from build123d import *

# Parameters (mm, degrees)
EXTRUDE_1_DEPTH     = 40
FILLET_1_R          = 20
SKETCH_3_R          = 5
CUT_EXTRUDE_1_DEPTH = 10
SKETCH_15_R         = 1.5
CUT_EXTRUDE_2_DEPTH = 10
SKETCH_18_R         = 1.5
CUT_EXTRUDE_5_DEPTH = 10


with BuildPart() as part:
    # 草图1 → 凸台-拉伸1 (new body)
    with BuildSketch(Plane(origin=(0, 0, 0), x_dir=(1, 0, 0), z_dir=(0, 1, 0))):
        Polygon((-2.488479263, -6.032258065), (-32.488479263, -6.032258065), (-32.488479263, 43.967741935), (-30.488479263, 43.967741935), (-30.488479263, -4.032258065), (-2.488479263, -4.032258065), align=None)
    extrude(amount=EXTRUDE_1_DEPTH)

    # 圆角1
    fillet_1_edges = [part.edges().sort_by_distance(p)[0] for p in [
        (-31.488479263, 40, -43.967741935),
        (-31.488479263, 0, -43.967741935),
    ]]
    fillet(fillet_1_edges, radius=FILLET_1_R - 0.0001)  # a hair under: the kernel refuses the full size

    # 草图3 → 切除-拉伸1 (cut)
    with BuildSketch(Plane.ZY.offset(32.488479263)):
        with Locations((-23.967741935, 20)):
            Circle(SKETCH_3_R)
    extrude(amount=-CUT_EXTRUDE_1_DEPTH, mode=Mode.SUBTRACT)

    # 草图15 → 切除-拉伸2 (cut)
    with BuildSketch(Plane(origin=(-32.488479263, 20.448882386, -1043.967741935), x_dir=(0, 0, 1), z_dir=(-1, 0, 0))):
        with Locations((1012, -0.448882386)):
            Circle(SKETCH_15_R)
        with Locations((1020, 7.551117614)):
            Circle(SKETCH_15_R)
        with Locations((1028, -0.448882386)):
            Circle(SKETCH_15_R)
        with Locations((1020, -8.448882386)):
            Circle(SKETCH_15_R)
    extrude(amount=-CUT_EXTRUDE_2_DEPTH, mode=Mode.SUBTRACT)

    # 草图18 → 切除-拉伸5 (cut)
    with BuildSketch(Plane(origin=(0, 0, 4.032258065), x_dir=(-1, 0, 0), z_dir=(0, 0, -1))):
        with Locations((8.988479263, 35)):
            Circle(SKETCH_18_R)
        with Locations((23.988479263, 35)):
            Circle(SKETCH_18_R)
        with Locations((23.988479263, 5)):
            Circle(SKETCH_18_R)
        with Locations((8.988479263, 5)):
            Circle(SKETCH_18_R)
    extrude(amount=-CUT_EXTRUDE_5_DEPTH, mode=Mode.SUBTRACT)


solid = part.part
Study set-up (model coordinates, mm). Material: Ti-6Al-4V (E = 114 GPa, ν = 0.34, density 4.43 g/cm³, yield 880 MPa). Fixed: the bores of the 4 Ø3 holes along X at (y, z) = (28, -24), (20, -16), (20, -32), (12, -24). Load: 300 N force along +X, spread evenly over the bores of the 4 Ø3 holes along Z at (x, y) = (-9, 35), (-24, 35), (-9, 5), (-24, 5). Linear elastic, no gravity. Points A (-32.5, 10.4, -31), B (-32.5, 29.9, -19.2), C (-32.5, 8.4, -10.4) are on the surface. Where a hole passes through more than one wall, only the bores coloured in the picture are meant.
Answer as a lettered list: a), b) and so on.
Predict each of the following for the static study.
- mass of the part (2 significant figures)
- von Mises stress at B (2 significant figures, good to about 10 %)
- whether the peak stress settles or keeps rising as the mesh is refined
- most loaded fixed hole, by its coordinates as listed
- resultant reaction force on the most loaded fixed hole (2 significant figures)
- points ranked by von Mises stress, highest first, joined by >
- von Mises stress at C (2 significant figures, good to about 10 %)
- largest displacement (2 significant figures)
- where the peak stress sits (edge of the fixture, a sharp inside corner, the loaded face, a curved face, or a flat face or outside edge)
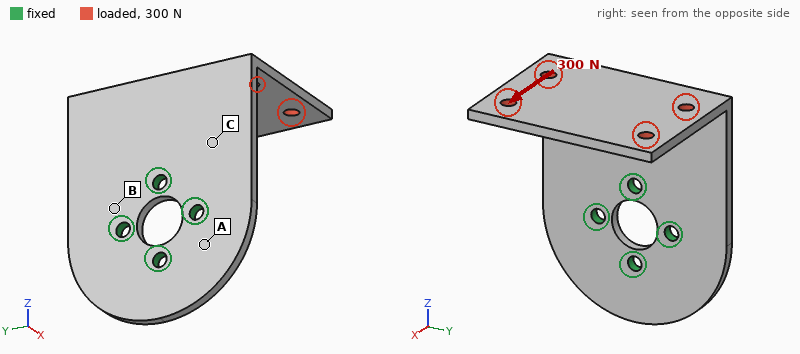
a) 25 g
b) 92 MPa
c) keeps rising
d) (20, -16)
e) 550 N
f) C > B > A
g) 140 MPa
h) 0.79 mm
i) edge of the fixture
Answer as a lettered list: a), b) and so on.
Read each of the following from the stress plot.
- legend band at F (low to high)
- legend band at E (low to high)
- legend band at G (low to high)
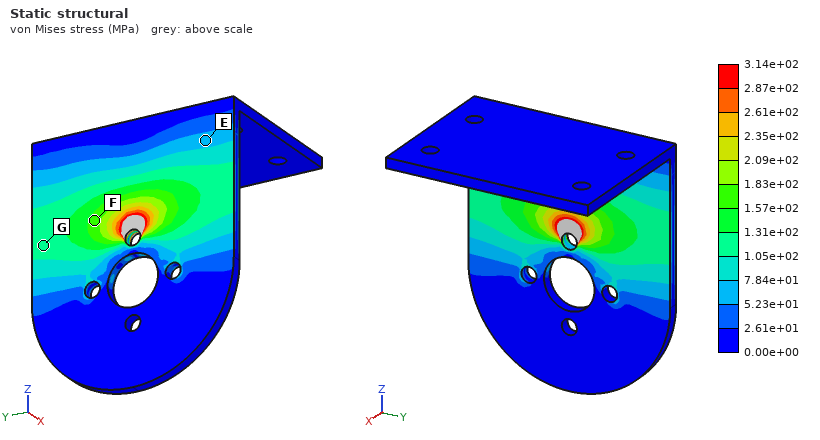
a) 1.57e+02 to 1.83e+02 MPa
b) 5.23e+01 to 7.84e+01 MPa
c) 1.05e+02 to 1.31e+02 MPa
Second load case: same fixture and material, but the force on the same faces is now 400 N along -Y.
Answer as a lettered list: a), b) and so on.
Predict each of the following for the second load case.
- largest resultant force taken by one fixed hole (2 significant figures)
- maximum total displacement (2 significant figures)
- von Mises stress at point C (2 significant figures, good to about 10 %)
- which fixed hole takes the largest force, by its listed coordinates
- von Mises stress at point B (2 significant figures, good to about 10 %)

a) 500 N
b) 0.80 mm
c) 110 MPa
d) (20, -16)
e) 150 MPa
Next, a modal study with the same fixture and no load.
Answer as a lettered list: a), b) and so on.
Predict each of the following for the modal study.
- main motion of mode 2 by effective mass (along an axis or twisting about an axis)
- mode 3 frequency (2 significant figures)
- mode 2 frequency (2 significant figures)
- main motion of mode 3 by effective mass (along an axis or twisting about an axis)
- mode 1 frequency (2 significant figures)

a) along Y
b) 2300 Hz
c) 1200 Hz
d) along X
e) 850 Hz
